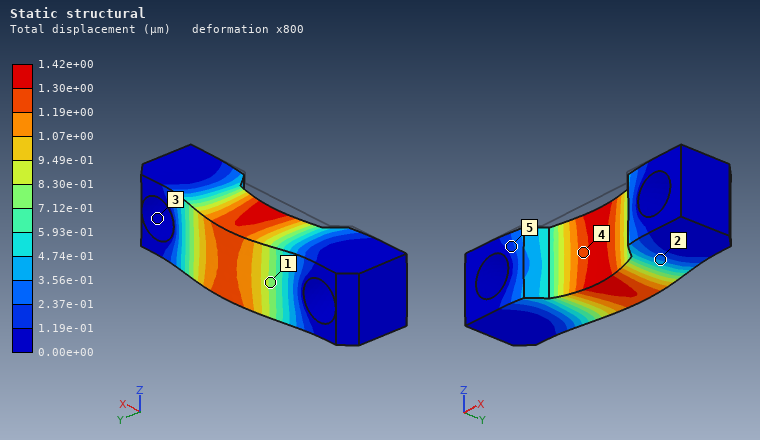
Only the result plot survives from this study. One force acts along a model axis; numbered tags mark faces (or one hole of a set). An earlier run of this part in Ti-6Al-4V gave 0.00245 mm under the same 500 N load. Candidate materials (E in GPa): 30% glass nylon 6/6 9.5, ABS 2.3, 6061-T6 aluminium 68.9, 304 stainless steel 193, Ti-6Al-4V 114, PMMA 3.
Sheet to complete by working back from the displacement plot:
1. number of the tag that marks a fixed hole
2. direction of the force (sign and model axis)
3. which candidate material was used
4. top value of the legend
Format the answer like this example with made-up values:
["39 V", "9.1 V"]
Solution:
["3", "+Y", "304 stainless steel", "1.42e+00 µm"]
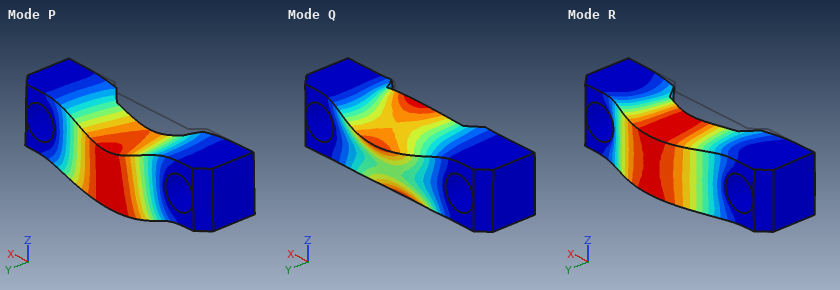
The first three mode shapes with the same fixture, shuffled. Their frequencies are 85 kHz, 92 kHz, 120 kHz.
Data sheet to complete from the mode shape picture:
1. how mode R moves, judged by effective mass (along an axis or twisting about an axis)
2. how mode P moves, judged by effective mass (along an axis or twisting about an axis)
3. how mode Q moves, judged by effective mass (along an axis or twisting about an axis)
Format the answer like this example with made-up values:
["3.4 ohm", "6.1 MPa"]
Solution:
["along Y", "along Z", "twisting about X"]
